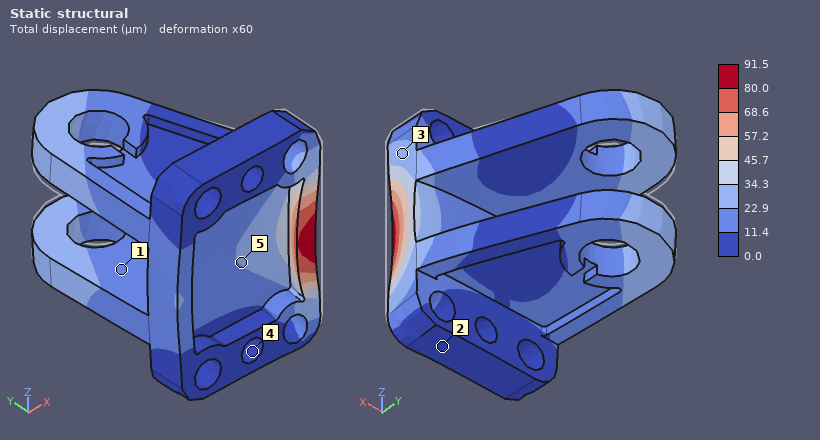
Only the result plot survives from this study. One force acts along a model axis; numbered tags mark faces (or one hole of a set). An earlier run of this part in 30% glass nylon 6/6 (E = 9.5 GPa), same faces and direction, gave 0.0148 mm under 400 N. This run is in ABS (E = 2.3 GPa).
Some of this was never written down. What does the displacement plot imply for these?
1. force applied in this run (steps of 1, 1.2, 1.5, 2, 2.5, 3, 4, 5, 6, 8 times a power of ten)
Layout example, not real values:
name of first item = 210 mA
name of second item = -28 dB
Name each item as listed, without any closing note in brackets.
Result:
force applied in this run = 600 N
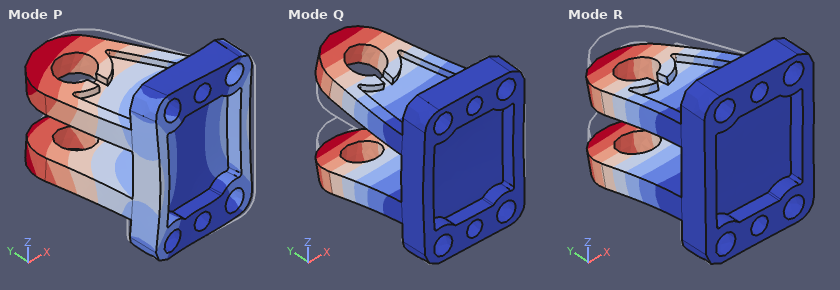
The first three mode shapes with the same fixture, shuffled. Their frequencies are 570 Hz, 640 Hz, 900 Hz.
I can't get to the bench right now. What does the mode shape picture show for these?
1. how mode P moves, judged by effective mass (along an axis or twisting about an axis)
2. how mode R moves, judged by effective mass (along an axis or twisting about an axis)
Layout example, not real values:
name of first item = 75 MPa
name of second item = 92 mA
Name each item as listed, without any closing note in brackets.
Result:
how mode P moves, judged by effective mass = along X
how mode R moves, judged by effective mass = along Z
